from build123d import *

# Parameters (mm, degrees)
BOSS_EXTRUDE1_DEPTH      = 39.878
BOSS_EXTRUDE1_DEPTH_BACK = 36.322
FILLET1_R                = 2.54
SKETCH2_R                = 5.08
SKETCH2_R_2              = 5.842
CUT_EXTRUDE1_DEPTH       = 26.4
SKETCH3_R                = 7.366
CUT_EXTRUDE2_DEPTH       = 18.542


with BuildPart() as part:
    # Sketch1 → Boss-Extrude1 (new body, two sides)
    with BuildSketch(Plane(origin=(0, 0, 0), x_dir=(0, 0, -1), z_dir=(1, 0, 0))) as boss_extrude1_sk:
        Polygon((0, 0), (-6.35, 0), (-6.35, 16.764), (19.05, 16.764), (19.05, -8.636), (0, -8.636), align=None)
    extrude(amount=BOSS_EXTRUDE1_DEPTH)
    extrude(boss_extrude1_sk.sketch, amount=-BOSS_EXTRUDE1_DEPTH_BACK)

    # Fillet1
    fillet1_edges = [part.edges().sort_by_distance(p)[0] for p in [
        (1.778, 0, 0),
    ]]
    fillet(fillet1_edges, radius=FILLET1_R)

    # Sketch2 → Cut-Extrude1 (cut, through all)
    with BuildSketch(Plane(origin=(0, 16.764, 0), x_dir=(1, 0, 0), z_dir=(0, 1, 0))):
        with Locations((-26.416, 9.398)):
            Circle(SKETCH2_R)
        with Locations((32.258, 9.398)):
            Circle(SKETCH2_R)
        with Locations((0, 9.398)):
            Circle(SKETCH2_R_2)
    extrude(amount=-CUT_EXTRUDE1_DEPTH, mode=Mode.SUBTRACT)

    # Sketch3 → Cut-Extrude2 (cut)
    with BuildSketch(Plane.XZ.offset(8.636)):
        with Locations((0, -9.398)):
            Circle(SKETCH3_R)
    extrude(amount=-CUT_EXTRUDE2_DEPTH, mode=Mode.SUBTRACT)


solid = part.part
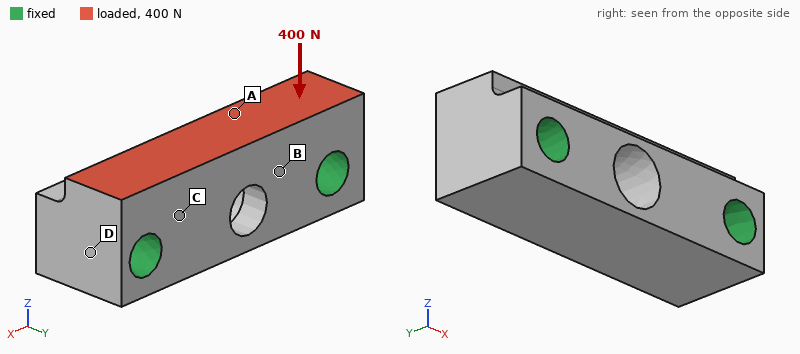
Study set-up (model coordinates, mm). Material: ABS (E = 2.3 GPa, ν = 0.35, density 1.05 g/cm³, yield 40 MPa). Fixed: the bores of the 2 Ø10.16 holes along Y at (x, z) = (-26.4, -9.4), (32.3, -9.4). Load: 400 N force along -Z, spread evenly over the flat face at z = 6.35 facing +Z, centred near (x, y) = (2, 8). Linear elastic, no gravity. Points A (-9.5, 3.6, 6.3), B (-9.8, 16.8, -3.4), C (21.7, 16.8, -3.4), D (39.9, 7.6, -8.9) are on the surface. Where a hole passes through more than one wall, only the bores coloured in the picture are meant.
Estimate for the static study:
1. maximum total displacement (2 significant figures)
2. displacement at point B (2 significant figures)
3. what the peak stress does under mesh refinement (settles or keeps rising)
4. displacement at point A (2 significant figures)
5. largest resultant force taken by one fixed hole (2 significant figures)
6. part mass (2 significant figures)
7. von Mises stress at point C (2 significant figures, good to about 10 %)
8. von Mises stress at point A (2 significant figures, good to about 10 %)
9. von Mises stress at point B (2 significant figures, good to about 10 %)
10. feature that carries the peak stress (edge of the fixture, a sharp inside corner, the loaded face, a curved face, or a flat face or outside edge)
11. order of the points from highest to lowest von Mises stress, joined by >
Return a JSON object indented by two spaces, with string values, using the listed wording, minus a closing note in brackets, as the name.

{
  "maximum total displacement": "12 µm",
  "displacement at point B": "7.1 µm",
  "what the peak stress does under mesh refinement": "keeps rising",
  "displacement at point A": "6.7 µm",
  "largest resultant force taken by one fixed hole": "210 N",
  "part mass": "39 g",
  "von Mises stress at point C": "0.64 MPa",
  "von Mises stress at point A": "0.29 MPa",
  "von Mises stress at point B": "0.47 MPa",
  "feature that carries the peak stress": "edge of the fixture",
  "order of the points from highest to lowest von Mises stress, joined by >": "C > B > A > D"
}
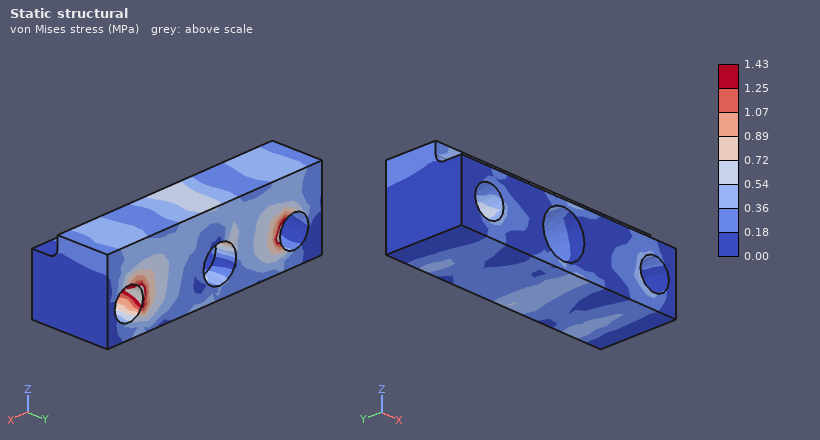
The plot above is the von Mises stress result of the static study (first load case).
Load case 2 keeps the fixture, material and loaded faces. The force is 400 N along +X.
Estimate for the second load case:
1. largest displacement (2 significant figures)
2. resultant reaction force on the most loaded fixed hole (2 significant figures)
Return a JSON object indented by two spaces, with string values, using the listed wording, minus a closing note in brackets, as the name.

{
  "largest displacement": "11 µm",
  "resultant reaction force on the most loaded fixed hole": "210 N"
}
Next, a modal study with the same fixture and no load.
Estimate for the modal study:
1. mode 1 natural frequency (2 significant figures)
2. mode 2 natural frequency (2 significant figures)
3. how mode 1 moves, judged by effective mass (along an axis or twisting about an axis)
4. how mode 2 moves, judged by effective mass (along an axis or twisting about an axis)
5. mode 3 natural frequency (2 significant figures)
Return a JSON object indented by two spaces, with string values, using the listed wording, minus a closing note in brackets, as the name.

{
  "mode 1 natural frequency": "6400 Hz",
  "mode 2 natural frequency": "6900 Hz",
  "how mode 1 moves, judged by effective mass": "along Z",
  "how mode 2 moves, judged by effective mass": "along Y",
  "mode 3 natural frequency": "8200 Hz"
}
